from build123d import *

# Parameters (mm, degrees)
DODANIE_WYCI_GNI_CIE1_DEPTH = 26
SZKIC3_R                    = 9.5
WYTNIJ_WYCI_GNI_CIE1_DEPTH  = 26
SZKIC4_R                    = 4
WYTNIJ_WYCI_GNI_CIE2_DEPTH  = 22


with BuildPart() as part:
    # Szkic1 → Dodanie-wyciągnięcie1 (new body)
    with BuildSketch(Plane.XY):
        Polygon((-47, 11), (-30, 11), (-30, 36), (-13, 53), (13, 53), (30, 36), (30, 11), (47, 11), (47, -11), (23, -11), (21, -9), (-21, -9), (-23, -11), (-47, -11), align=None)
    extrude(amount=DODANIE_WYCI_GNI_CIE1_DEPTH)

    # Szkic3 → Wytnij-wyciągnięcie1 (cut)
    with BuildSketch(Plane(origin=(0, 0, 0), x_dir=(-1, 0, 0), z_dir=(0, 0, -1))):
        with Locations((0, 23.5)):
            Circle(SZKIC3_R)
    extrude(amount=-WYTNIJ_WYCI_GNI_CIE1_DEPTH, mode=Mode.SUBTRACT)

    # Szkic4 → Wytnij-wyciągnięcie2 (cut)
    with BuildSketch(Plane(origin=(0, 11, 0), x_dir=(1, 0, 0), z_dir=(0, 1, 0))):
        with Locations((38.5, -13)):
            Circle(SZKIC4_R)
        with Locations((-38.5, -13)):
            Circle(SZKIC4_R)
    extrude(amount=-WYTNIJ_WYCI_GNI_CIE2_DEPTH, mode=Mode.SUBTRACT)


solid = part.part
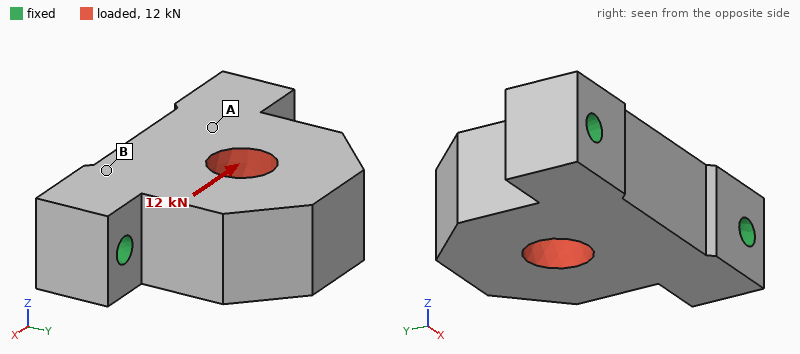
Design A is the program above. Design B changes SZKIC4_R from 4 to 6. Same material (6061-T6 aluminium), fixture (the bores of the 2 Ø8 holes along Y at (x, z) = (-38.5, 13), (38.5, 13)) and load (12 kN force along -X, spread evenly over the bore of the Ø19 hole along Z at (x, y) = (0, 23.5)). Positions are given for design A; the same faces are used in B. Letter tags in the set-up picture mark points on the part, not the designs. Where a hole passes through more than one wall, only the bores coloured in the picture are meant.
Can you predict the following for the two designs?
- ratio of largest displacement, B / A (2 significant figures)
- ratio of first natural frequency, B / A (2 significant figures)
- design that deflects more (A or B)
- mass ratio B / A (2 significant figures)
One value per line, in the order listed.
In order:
0.89
1.1
A
0.97
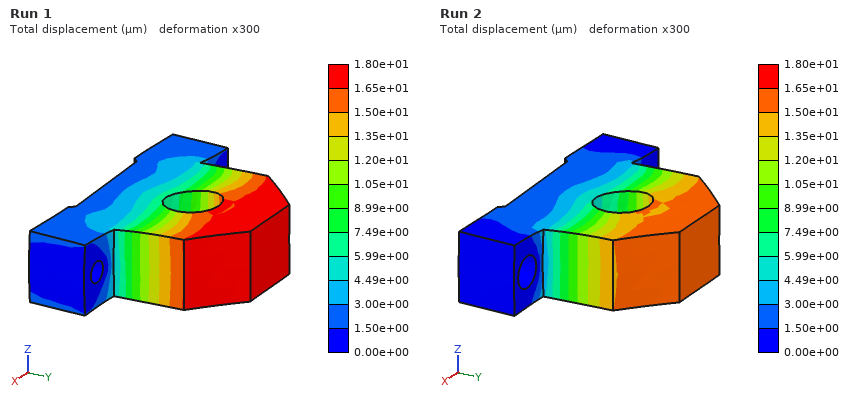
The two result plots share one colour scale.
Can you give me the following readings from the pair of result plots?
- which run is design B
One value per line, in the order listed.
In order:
Run 2
